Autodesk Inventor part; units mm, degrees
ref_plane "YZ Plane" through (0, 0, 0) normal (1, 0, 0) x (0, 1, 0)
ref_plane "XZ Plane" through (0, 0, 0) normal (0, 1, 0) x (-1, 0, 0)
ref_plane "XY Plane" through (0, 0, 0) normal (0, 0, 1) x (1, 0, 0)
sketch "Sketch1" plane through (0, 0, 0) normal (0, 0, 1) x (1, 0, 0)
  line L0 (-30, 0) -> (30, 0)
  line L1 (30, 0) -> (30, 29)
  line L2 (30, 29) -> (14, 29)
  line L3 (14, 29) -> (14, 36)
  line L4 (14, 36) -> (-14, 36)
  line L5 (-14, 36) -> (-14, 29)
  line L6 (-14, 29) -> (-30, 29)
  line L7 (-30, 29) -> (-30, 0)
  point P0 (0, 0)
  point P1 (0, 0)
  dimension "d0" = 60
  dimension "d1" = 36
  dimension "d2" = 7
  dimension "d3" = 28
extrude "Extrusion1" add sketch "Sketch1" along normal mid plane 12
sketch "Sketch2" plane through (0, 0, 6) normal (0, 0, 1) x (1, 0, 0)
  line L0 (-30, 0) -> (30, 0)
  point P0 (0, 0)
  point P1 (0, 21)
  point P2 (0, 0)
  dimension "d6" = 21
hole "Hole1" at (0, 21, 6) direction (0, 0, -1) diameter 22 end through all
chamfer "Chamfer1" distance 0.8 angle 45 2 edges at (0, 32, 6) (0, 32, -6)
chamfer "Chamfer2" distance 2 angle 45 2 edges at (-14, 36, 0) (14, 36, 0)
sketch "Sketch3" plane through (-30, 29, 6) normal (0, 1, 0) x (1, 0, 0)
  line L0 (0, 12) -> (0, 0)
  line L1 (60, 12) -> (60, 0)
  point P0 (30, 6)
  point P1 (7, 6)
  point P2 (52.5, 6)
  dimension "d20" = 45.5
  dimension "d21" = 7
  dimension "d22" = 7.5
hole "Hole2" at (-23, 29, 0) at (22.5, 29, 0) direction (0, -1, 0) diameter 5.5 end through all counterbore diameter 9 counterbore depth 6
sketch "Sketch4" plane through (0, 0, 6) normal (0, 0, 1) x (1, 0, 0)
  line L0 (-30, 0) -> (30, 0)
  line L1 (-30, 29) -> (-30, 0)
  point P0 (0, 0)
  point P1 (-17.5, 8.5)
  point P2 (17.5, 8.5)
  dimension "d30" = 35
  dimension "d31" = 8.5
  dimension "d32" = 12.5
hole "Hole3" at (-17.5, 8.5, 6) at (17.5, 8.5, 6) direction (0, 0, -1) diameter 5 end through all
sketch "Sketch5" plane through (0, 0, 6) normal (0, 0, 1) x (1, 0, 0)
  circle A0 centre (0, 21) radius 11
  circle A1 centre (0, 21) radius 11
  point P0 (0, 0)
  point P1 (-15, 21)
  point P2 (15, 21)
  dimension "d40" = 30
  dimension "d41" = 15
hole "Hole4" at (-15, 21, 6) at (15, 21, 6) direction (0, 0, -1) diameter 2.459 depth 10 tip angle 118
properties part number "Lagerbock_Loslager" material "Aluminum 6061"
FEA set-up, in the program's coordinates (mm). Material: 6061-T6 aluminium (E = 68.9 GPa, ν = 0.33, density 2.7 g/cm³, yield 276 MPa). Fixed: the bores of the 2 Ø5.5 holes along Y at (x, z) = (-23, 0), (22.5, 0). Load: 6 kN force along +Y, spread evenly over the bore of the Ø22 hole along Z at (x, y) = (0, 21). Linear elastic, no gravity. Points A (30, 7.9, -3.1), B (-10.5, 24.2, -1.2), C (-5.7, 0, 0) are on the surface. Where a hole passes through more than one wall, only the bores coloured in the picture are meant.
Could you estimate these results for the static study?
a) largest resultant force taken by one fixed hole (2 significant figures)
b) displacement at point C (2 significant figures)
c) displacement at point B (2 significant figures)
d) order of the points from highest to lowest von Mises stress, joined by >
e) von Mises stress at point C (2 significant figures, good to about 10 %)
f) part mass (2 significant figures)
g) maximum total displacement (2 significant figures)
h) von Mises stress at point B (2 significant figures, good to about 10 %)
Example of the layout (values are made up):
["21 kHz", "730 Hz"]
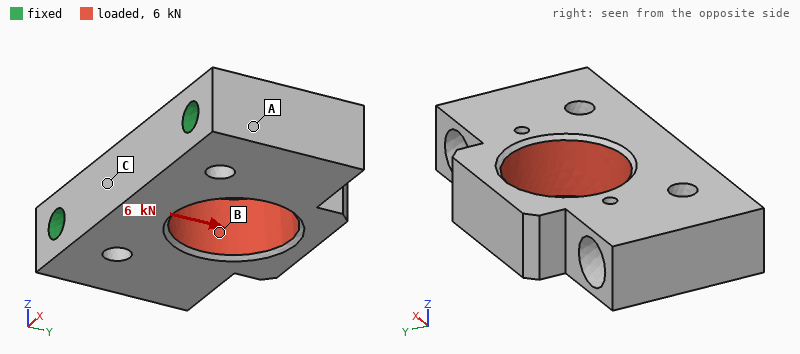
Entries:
["3.1 kN", "6.6 µm", "7.6 µm", "B > C > A", "11 MPa", "44 g", "14 µm", "28 MPa"]
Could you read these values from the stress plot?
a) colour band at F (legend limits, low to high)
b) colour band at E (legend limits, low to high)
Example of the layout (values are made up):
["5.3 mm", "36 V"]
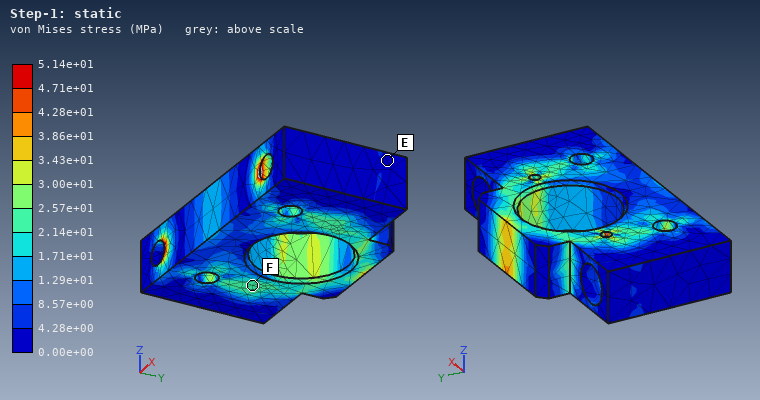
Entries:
["2.14e+01 to 2.57e+01 MPa", "0.00e+00 to 4.28e+00 MPa"]
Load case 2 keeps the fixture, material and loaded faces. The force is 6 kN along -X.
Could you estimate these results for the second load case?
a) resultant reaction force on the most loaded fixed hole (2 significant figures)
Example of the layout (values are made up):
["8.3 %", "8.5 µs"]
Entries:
["3.0 kN"]
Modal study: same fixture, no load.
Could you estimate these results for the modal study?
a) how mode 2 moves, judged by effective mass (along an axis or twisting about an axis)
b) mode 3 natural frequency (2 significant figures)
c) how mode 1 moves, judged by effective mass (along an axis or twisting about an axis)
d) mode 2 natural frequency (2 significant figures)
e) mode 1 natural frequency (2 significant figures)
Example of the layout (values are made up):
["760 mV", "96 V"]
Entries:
["along Z", "27 kHz", "along Z", "22 kHz", "15 kHz"]
